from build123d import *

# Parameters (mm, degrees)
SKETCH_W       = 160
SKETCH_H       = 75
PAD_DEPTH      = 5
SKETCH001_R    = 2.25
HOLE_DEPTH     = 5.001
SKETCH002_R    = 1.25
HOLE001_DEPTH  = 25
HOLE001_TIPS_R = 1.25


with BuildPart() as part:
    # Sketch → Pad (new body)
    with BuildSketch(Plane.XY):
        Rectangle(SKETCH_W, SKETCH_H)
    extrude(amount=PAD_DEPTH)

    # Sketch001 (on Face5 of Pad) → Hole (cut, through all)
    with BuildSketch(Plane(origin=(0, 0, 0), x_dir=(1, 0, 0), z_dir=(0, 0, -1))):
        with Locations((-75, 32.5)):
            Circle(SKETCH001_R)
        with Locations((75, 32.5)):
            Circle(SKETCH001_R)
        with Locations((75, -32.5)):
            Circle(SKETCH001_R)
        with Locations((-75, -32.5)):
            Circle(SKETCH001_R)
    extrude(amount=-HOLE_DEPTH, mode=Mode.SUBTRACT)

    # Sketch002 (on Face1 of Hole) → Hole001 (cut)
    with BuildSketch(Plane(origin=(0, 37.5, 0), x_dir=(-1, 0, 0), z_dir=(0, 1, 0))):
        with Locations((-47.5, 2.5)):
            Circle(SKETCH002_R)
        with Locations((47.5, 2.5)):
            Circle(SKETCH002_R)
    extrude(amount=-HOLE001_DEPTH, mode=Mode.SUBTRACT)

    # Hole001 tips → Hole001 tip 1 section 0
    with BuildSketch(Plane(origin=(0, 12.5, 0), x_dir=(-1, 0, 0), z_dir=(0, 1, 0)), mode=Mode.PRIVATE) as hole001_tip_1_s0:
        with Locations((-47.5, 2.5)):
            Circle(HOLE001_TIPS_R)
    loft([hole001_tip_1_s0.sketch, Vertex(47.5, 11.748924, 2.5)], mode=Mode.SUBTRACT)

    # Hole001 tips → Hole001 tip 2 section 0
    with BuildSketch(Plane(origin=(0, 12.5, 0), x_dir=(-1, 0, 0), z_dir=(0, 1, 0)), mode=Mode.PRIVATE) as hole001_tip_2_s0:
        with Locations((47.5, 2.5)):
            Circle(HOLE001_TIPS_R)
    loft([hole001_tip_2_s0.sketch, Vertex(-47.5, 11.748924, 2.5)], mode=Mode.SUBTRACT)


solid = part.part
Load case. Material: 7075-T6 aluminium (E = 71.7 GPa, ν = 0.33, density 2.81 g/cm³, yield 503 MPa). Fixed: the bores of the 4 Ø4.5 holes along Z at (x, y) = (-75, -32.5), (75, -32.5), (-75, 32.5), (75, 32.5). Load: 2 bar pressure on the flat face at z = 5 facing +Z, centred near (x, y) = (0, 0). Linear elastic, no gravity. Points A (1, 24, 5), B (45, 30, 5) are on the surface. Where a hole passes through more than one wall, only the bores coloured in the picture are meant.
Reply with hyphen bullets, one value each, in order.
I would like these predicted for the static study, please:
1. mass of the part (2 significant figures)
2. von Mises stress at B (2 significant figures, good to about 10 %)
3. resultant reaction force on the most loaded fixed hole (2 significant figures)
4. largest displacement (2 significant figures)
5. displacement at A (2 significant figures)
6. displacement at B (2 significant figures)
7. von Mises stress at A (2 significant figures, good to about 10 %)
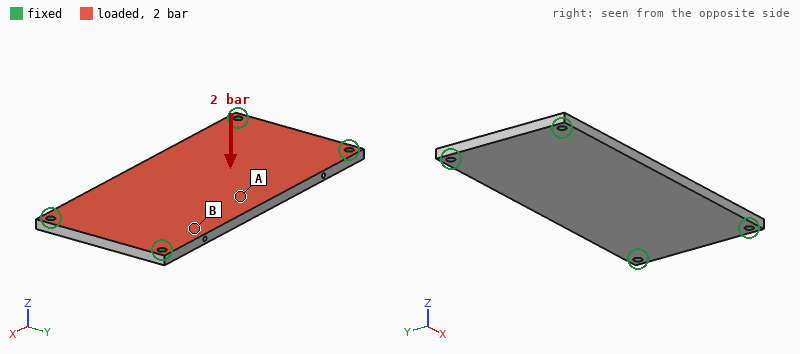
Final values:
- 170 g
- 22 MPa
- 600 N
- 0.51 mm
- 0.49 mm
- 0.23 mm
- 53 MPa
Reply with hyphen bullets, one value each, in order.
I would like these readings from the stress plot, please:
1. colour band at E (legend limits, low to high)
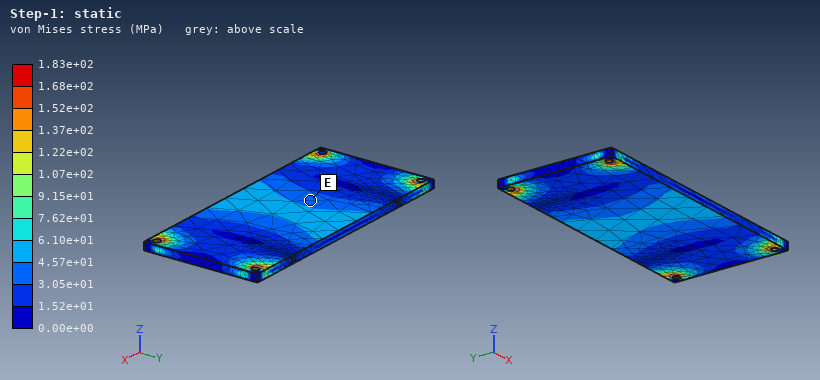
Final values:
- 3.05e+01 to 4.57e+01 MPa
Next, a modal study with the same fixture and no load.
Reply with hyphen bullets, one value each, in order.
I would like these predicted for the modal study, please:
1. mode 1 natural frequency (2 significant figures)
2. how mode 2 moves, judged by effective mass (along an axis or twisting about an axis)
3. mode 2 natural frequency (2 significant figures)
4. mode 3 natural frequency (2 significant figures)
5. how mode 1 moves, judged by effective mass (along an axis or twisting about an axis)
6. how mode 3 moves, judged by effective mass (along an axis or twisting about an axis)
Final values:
- 980 Hz
- twisting about X
- 1900 Hz
- 2700 Hz
- along Z
- twisting about Y
